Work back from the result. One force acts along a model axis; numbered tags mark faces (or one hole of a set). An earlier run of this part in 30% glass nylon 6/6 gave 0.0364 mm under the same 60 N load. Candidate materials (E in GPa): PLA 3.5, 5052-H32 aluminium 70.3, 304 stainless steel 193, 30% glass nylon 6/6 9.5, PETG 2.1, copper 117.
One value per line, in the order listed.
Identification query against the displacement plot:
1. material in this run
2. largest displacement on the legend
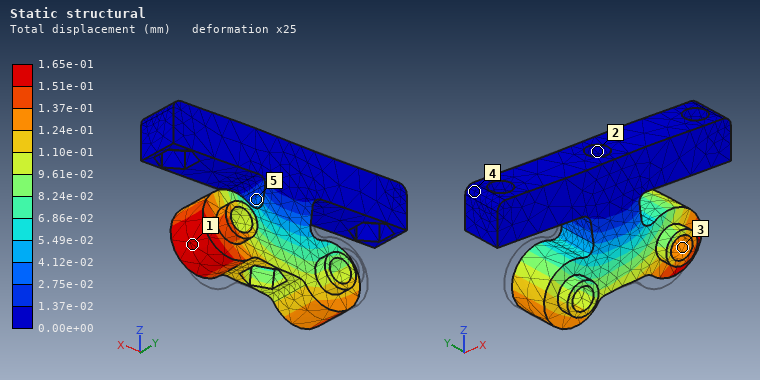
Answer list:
PETG
1.65e-01 mm
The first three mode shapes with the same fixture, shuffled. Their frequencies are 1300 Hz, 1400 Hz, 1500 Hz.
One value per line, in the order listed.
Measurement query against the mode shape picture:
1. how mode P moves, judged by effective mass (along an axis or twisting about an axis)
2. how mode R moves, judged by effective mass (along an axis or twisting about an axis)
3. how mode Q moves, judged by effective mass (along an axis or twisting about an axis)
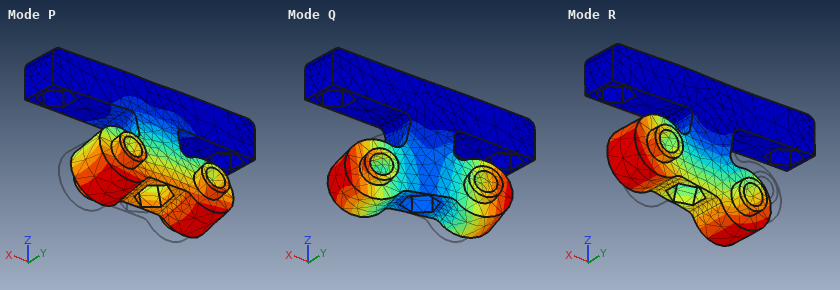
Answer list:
along Y
along X
twisting about Z
